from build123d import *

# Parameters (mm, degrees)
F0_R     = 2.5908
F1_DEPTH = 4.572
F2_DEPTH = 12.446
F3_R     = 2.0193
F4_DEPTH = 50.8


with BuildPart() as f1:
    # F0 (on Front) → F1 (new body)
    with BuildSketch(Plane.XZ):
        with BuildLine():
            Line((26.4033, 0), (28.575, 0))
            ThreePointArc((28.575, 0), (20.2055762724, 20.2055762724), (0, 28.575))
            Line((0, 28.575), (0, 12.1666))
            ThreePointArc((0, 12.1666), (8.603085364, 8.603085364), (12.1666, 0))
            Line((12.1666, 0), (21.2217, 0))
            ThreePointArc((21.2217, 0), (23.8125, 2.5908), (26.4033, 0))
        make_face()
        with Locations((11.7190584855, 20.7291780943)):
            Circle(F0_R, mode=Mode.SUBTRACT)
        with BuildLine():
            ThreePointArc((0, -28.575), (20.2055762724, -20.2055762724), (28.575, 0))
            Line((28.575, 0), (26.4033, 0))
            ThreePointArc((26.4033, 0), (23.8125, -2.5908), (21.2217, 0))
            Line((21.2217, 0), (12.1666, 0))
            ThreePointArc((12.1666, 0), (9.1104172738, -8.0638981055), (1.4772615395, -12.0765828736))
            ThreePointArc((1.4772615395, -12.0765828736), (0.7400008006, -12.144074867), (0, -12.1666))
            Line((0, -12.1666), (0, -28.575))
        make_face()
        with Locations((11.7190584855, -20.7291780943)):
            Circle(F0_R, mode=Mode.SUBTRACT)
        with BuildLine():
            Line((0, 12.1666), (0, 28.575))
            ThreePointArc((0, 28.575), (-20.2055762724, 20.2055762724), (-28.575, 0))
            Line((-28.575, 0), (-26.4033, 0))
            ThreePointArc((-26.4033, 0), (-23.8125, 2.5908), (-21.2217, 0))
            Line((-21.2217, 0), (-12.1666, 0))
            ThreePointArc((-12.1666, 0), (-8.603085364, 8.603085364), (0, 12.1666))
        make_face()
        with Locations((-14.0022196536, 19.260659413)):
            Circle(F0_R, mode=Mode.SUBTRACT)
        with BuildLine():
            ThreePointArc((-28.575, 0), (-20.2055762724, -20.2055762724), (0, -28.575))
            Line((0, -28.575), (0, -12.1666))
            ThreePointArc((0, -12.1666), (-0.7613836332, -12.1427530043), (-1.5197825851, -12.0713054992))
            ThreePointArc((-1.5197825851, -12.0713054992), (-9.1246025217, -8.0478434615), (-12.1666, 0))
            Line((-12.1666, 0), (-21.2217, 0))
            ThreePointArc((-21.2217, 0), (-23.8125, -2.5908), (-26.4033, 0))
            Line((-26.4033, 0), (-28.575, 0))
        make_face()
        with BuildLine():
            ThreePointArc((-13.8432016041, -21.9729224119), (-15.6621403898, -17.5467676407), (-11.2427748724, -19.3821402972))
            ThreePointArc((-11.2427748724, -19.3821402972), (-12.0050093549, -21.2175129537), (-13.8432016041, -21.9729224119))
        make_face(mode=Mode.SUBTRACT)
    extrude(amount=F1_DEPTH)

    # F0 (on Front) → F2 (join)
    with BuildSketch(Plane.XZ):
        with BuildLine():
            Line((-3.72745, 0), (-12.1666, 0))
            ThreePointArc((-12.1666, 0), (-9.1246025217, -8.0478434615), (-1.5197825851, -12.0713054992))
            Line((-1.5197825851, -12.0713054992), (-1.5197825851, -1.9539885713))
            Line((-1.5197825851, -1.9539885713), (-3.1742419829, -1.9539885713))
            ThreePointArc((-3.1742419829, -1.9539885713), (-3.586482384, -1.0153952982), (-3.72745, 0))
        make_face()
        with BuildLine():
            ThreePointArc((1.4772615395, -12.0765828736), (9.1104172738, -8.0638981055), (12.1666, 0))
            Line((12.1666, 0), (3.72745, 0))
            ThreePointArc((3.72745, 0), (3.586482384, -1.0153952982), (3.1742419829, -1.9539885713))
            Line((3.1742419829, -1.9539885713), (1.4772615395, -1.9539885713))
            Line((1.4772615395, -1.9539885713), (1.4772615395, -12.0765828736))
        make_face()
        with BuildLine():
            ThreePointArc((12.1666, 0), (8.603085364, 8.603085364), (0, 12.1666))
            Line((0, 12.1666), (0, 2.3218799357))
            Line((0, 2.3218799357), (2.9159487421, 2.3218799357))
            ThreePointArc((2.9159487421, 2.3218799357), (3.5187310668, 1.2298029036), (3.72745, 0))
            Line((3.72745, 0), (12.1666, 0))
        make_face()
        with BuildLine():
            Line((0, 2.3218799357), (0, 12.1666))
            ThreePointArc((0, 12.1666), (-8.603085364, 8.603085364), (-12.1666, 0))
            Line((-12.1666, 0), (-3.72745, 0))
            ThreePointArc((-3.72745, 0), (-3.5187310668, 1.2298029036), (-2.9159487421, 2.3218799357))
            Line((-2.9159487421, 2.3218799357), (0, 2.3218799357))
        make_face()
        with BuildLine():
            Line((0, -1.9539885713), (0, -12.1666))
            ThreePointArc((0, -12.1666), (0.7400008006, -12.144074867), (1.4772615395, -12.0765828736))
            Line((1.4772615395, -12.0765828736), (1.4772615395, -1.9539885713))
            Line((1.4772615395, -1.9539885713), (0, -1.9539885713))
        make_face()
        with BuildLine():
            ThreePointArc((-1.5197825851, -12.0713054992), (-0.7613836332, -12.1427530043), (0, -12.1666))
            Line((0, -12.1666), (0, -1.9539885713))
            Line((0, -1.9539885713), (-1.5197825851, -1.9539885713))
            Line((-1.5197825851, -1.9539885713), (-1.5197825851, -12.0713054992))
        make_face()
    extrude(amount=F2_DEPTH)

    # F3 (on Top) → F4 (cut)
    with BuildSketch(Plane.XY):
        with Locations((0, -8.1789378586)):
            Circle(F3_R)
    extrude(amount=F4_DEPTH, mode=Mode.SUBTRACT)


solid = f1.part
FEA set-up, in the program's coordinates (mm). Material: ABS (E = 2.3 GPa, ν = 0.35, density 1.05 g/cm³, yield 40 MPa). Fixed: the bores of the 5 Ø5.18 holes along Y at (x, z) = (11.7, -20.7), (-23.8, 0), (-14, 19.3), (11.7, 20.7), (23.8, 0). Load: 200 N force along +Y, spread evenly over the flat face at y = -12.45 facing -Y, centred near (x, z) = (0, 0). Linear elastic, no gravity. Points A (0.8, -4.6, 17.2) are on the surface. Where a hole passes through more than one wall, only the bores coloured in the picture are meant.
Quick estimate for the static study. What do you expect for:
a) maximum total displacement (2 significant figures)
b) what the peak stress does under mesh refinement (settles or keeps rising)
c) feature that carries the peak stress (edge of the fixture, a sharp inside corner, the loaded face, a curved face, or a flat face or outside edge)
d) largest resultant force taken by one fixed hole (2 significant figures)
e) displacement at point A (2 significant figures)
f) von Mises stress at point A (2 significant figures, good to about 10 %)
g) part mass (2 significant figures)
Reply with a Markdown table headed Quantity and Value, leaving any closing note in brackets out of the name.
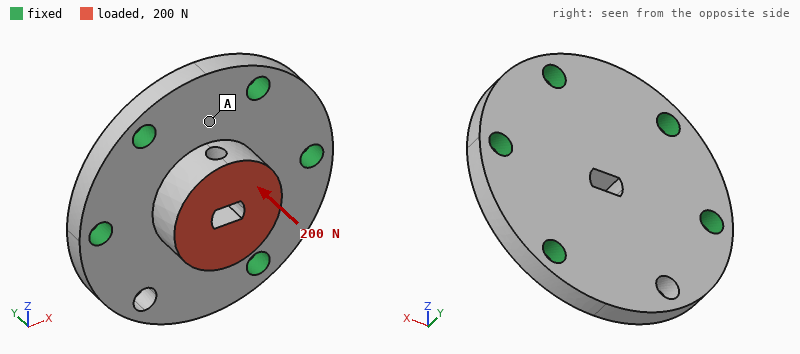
| Quantity | Value |
|---|---|
| maximum total displacement | 46 µm |
| what the peak stress does under mesh refinement | keeps rising |
| feature that carries the peak stress | edge of the fixture |
| largest resultant force taken by one fixed hole | 54 N |
| displacement at point A | 15 µm |
| von Mises stress at point A | 0.93 MPa |
| part mass | 15 g |
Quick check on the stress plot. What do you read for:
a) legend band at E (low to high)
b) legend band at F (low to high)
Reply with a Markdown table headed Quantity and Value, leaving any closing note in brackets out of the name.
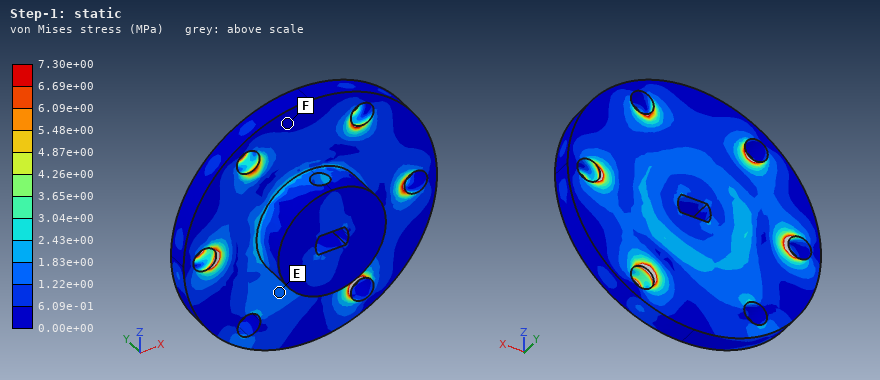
| Quantity | Value |
|---|---|
| legend band at E | 1.22e+00 to 1.83e+00 MPa |
| legend band at F | 0.00e+00 to 6.09e-01 MPa |
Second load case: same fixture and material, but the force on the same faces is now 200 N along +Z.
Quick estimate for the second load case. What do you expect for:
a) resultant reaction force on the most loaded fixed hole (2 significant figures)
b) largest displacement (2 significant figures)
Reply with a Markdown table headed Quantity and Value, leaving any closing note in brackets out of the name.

| Quantity | Value |
|---|---|
| resultant reaction force on the most loaded fixed hole | 74 N |
| largest displacement | 51 µm |
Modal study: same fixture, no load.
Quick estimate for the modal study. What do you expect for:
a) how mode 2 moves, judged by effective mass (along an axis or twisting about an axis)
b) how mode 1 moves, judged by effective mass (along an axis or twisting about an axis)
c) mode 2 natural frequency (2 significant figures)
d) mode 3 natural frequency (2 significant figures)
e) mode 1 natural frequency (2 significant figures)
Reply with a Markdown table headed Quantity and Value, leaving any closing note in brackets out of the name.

| Quantity | Value |
|---|---|
| how mode 2 moves, judged by effective mass | along Y |
| how mode 1 moves, judged by effective mass | along Y |
| mode 2 natural frequency | 4900 Hz |
| mode 3 natural frequency | 6900 Hz |
| mode 1 natural frequency | 3300 Hz |
